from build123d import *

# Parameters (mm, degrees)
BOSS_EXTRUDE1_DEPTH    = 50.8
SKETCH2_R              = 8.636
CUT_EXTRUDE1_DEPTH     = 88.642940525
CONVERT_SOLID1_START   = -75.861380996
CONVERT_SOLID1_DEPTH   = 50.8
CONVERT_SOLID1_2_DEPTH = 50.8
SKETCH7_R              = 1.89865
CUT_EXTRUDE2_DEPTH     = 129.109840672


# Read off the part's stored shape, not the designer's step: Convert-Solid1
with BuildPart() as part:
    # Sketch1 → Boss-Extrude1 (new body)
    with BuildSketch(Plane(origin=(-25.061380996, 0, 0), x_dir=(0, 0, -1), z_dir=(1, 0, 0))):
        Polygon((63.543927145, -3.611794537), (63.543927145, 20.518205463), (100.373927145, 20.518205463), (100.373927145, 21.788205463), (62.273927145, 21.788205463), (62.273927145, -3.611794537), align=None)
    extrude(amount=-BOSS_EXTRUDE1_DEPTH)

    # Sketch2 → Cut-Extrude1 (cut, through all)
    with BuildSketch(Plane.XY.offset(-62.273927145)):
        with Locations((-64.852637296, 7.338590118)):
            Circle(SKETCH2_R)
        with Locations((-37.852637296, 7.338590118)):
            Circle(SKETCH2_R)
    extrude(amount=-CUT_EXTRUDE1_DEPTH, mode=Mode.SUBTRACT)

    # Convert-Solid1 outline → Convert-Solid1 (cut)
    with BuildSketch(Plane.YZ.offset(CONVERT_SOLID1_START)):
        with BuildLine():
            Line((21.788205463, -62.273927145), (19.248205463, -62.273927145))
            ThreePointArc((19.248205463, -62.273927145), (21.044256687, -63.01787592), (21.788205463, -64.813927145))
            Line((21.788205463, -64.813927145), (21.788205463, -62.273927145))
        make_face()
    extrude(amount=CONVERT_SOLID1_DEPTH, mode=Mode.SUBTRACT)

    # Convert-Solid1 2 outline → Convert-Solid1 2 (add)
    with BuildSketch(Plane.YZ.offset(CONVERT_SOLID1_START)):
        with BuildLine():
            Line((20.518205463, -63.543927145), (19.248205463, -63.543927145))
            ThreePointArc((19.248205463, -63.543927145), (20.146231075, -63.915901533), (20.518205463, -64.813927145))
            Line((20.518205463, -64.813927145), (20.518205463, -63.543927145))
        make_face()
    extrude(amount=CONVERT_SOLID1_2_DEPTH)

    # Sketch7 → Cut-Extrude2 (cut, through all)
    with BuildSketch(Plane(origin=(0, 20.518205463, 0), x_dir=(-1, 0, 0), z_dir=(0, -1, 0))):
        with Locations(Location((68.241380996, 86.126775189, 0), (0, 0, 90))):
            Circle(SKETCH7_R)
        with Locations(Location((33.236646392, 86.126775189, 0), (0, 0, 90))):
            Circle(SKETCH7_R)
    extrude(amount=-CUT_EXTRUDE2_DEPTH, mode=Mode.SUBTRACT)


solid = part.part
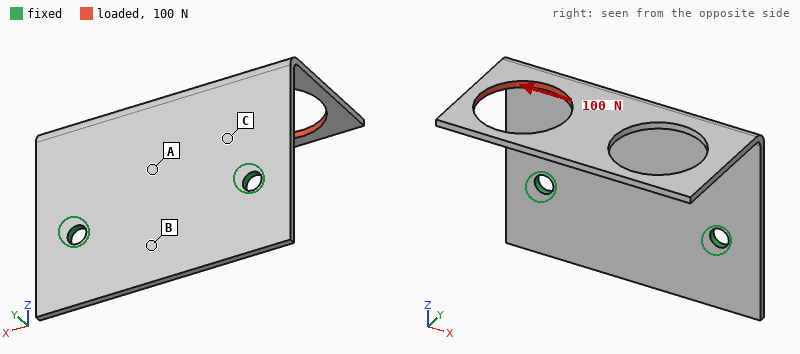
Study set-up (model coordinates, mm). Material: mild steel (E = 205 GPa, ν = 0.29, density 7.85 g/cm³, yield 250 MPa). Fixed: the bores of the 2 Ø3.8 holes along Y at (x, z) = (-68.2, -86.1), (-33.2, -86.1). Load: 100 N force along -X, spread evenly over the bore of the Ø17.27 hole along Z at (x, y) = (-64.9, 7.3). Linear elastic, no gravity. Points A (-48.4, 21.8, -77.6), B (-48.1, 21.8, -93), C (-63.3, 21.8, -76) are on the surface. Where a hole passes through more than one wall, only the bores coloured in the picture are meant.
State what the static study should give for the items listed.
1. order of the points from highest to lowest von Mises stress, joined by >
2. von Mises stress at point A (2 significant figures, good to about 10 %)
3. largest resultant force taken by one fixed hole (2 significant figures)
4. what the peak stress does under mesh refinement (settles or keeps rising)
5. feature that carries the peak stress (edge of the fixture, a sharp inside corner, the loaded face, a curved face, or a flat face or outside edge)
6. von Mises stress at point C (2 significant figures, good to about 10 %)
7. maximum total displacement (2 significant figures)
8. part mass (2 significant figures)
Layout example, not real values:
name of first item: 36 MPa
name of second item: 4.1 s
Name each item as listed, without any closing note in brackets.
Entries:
order of the points from highest to lowest von Mises stress, joined by >: C > A > B
von Mises stress at point A: 29 MPa
largest resultant force taken by one fixed hole: 88 N
what the peak stress does under mesh refinement: keeps rising
feature that carries the peak stress: edge of the fixture
von Mises stress at point C: 45 MPa
maximum total displacement: 0.18 mm
part mass: 26 g
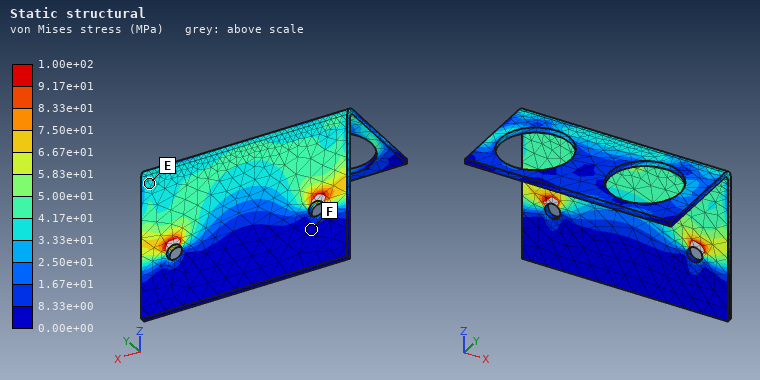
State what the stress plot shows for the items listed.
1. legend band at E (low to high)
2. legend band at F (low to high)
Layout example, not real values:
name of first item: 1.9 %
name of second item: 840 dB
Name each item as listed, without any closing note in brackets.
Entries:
legend band at E: 3.33e+01 to 4.17e+01 MPa
legend band at F: 0.00e+00 to 8.33e+00 MPa
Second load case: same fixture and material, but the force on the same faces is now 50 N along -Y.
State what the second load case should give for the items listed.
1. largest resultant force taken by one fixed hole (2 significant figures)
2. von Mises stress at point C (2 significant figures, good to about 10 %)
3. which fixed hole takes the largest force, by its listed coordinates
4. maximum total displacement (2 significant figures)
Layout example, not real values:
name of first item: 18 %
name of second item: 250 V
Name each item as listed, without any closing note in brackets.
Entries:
largest resultant force taken by one fixed hole: 44 N
von Mises stress at point C: 62 MPa
which fixed hole takes the largest force, by its listed coordinates: (-68.2, -86.1)
maximum total displacement: 0.30 mm
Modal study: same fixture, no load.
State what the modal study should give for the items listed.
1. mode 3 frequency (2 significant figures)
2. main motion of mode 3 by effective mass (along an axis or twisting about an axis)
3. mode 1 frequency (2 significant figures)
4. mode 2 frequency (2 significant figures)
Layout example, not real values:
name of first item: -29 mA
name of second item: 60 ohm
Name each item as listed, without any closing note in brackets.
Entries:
mode 3 frequency: 1700 Hz
main motion of mode 3 by effective mass: along Y
mode 1 frequency: 740 Hz
mode 2 frequency: 1300 Hz
